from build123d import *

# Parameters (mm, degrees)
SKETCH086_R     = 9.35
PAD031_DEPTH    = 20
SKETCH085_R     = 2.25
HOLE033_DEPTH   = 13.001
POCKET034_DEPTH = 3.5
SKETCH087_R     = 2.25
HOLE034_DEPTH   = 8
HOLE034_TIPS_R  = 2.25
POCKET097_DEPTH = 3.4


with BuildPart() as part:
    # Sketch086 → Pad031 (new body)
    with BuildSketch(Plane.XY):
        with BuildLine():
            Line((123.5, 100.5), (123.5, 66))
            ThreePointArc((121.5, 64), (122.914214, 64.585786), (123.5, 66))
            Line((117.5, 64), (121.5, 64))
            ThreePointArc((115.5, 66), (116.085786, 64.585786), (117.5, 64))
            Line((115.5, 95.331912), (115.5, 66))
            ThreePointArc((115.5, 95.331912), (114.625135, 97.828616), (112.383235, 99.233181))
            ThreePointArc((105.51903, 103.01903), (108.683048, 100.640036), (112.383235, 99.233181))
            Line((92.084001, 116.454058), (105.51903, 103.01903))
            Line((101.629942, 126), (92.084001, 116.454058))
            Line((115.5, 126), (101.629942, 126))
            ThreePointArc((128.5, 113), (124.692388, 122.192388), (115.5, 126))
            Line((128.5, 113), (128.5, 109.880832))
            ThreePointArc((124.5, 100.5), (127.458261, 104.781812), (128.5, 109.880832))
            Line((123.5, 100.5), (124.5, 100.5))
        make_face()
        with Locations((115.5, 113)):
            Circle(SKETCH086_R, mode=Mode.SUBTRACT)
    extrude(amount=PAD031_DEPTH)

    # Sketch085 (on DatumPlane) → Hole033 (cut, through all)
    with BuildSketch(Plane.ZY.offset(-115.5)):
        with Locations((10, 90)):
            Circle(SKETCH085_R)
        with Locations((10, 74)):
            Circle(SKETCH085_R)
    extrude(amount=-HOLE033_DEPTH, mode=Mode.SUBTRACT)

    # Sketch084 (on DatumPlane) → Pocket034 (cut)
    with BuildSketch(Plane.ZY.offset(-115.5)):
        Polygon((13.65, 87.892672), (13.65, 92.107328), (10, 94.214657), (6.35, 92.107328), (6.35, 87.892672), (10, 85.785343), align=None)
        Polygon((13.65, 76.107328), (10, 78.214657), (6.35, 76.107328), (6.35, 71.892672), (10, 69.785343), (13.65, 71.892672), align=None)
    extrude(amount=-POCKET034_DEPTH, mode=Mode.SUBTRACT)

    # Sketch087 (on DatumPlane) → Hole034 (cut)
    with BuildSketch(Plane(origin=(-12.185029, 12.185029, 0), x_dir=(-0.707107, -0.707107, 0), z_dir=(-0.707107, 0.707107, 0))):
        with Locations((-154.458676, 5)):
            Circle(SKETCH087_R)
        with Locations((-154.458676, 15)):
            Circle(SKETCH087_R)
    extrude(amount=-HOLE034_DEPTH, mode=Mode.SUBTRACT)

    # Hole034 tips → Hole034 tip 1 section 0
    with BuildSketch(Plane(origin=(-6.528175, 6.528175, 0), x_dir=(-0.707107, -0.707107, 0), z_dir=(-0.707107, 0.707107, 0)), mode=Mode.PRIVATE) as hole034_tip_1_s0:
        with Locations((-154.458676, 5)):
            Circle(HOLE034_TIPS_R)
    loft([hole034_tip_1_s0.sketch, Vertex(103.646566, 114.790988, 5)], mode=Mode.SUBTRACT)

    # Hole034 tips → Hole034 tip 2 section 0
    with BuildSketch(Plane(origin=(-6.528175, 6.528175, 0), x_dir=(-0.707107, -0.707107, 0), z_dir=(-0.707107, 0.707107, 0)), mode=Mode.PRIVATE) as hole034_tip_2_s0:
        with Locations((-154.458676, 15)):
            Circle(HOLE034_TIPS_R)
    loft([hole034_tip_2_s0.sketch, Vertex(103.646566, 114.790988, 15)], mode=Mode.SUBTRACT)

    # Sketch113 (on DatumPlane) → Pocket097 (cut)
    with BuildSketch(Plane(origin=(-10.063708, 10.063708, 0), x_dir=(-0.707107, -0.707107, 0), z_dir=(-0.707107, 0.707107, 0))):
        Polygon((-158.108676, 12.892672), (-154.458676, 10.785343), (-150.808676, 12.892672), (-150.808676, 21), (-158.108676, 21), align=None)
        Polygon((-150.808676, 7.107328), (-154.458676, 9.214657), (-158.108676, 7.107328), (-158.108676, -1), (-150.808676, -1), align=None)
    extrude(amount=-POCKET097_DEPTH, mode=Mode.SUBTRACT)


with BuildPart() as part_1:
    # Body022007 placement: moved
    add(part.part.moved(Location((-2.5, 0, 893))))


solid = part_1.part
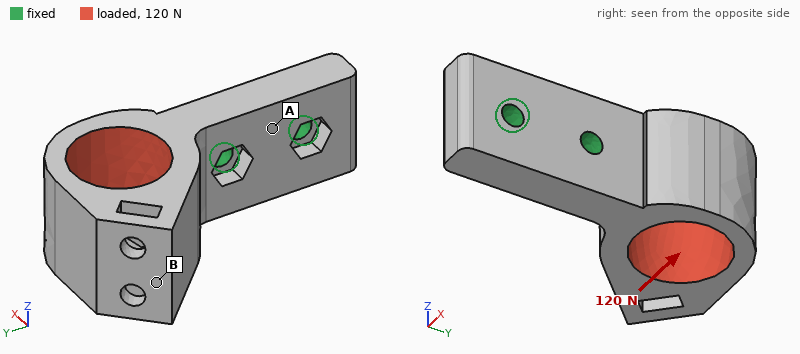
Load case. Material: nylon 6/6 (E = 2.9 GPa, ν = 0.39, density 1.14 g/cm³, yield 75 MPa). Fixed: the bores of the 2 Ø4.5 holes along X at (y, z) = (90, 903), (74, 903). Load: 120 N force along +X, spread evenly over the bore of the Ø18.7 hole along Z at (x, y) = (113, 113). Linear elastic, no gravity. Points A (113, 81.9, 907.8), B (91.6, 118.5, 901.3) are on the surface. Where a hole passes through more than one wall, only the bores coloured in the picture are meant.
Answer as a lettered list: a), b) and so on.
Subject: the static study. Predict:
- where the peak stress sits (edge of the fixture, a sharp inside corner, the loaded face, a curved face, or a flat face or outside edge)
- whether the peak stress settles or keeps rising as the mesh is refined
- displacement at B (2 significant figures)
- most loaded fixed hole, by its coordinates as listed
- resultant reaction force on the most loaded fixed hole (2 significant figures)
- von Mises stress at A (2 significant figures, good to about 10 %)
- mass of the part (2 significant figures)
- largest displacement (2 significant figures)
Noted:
a) edge of the fixture
b) keeps rising
c) 0.63 mm
d) (90, 903)
e) 240 N
f) 3.9 MPa
g) 16 g
h) 0.65 mm
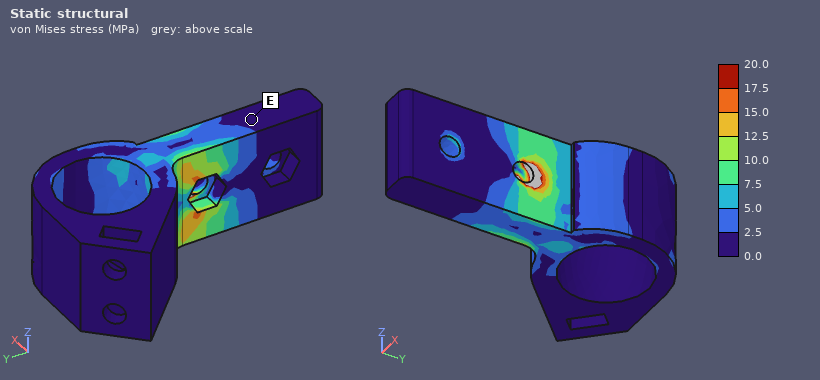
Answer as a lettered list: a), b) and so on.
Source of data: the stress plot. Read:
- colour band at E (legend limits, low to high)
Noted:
a) 0.0 to 2.5 MPa
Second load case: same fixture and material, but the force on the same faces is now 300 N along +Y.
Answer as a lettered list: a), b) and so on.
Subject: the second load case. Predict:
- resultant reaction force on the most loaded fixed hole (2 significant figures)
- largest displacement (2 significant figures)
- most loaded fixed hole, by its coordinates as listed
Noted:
a) 180 N
b) 0.40 mm
c) (90, 903)
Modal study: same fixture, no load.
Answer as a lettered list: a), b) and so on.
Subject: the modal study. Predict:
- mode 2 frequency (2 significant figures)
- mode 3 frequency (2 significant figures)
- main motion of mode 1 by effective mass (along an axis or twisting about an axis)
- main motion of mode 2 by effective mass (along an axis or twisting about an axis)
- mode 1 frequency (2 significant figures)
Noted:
a) 1200 Hz
b) 2300 Hz
c) along X
d) along Z
e) 750 Hz
